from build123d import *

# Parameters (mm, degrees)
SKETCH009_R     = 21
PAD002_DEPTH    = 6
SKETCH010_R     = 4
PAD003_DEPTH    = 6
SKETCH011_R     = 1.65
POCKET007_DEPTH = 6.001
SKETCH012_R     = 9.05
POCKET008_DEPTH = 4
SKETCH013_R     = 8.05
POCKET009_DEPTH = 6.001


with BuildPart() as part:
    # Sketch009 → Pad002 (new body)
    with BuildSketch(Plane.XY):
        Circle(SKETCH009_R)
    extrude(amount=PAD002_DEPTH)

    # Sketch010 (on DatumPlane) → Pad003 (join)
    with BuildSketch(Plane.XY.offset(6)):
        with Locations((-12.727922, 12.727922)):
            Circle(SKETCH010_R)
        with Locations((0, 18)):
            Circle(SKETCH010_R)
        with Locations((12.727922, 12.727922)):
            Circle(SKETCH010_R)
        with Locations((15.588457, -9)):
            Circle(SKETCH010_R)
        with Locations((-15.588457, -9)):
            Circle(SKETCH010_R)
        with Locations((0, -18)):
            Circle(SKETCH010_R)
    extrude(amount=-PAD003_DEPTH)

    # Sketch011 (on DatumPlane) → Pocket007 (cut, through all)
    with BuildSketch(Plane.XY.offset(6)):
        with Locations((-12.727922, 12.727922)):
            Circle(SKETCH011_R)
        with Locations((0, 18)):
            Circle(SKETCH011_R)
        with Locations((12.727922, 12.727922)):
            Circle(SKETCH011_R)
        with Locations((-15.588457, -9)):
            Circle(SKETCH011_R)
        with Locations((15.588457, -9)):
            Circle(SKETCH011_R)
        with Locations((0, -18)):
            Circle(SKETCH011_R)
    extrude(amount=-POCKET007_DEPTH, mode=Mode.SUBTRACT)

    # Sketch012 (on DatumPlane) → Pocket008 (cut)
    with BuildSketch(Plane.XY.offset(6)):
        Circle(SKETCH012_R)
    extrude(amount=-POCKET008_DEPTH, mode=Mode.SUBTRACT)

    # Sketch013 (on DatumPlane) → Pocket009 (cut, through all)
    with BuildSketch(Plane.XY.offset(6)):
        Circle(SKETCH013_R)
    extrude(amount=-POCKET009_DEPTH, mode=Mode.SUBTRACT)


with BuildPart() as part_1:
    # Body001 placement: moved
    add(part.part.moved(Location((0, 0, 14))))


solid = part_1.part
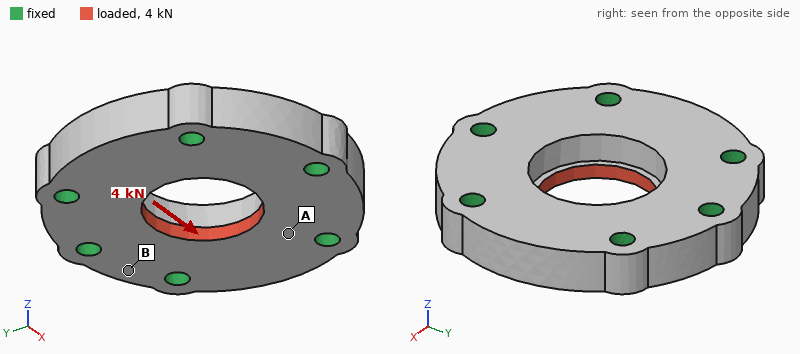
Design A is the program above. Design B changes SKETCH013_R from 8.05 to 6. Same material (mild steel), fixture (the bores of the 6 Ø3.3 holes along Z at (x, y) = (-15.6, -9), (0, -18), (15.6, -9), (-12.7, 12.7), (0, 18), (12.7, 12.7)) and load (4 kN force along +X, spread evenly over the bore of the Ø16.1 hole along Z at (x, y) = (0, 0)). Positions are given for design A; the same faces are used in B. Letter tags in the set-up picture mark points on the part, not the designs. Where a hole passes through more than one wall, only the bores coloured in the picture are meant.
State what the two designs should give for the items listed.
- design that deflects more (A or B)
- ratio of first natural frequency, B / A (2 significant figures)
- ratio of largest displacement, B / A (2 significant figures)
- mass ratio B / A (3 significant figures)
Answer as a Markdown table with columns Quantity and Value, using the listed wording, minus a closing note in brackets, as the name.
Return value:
| Quantity | Value |
|---|---|
| design that deflects more | B |
| ratio of first natural frequency, B / A | 0.94 |
| ratio of largest displacement, B / A | 1.3 |
| mass ratio B / A | 1.03 |
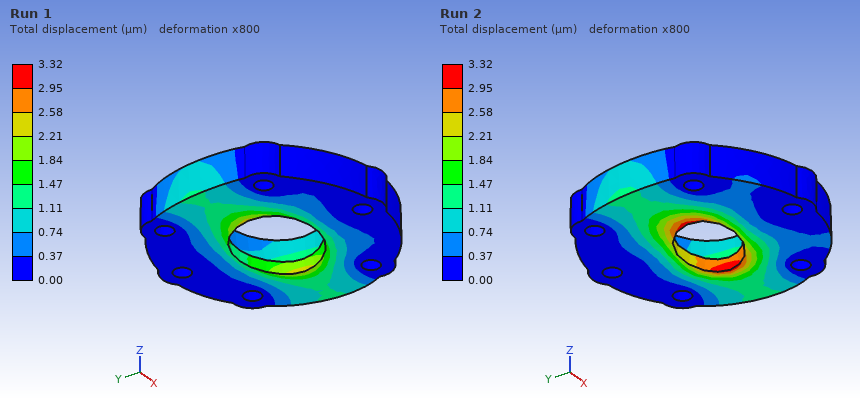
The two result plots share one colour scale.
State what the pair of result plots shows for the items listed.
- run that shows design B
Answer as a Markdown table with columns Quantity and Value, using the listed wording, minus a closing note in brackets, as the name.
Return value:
| Quantity | Value |
|---|---|
| run that shows design B | Run 2 |
